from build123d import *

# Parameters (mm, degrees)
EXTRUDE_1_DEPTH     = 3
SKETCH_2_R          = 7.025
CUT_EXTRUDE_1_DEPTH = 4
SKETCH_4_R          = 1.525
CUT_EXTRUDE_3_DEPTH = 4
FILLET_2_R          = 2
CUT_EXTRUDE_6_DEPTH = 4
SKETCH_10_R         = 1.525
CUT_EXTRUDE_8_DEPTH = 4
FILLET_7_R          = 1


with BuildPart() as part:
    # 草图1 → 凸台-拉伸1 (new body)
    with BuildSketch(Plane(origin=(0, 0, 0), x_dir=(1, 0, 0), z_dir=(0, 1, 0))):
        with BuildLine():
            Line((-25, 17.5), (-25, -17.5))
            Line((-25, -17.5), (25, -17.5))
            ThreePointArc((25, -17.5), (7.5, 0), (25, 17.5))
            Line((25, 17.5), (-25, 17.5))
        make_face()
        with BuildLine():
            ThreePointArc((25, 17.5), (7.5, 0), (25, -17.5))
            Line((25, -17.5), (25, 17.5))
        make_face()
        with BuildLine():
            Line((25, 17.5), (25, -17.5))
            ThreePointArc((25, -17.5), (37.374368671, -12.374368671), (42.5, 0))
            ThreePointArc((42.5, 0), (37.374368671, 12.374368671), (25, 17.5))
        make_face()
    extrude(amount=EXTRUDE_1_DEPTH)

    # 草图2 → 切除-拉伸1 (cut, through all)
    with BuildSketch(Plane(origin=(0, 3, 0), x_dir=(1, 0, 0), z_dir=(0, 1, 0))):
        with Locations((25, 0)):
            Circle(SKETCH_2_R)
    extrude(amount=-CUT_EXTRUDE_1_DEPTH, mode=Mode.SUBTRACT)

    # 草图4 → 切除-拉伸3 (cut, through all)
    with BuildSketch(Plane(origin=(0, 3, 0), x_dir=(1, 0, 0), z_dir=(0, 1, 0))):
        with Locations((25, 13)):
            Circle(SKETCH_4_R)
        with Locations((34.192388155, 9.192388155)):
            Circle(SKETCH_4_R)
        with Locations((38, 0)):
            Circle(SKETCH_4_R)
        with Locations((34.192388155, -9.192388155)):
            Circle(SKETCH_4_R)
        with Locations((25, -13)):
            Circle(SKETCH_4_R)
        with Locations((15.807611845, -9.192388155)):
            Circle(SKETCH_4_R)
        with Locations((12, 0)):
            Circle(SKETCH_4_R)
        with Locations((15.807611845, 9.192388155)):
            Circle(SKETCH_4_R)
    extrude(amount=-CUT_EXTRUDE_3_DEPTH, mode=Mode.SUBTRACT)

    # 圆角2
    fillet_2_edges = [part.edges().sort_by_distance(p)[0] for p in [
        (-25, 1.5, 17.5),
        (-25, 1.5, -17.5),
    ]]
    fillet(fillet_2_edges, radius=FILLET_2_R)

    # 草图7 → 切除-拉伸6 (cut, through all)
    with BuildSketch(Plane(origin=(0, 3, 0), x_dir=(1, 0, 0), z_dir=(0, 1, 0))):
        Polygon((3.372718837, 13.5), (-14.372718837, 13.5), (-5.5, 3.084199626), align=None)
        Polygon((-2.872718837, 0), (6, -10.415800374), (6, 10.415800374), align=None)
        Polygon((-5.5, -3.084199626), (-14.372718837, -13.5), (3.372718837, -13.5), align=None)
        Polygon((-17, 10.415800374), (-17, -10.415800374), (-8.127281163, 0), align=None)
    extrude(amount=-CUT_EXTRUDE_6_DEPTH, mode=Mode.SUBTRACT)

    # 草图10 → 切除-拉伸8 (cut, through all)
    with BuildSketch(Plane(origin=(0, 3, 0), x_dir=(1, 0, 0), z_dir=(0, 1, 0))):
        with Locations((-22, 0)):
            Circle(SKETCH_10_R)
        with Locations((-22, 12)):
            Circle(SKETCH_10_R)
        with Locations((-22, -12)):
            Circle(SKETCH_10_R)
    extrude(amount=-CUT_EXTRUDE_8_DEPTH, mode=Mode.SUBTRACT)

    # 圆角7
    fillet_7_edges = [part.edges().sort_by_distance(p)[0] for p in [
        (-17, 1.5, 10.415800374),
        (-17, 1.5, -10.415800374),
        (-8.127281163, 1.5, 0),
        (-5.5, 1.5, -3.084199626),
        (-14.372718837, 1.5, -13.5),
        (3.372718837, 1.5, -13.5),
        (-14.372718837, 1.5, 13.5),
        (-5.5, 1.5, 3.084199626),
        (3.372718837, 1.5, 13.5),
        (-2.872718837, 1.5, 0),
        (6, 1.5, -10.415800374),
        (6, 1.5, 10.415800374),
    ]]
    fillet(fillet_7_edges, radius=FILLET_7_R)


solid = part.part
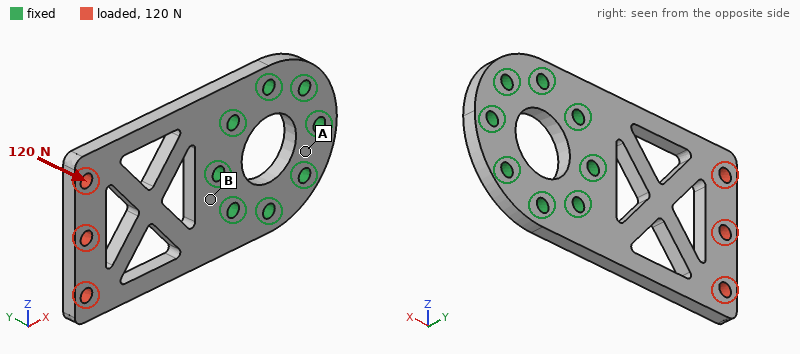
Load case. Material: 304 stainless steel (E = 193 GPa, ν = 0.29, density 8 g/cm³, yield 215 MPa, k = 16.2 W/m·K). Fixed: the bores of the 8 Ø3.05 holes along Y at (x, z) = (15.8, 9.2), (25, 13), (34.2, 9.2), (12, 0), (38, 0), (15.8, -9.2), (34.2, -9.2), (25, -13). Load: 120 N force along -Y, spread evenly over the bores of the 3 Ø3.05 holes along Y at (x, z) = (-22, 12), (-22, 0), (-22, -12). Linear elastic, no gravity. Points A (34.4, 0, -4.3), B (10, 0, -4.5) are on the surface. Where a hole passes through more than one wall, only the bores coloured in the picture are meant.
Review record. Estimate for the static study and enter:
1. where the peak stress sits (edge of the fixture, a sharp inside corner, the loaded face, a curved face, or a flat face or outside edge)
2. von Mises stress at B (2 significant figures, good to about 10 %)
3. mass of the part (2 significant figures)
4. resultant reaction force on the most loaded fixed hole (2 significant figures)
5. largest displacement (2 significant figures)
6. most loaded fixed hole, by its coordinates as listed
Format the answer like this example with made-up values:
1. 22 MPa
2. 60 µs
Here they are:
1. a curved face
2. 59 MPa
3. 39 g
4. 150 N
5. 0.27 mm
6. (12, 0)
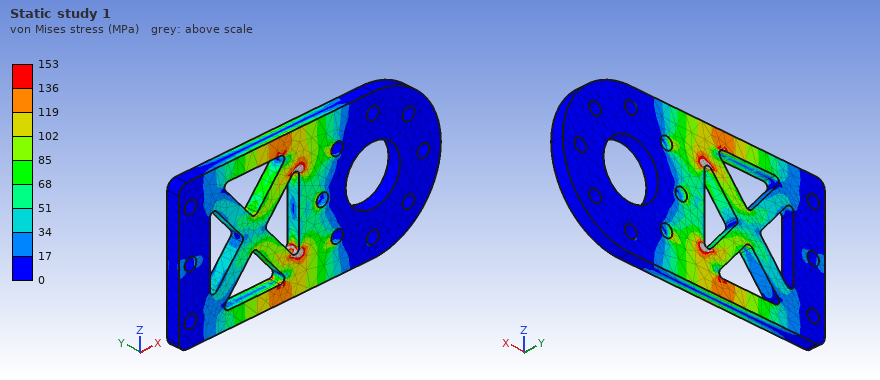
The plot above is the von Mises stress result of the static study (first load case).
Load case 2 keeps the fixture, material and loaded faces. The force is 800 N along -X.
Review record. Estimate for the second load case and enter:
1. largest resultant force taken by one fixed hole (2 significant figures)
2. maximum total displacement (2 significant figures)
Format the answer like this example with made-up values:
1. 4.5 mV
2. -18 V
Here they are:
1. 280 N
2. 9.6 µm
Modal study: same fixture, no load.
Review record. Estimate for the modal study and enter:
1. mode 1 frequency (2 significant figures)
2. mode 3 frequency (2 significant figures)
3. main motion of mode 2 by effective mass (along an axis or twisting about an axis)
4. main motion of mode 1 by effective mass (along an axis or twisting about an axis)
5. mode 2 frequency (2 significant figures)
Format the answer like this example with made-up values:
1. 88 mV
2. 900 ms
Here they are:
1. 1300 Hz
2. 7900 Hz
3. twisting about X
4. along Y
5. 3200 Hz
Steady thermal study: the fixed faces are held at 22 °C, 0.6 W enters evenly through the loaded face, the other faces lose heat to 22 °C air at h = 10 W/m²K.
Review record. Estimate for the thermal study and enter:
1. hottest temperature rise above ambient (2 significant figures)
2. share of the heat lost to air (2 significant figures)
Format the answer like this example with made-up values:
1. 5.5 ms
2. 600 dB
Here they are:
1. 20 K
2. 43 %
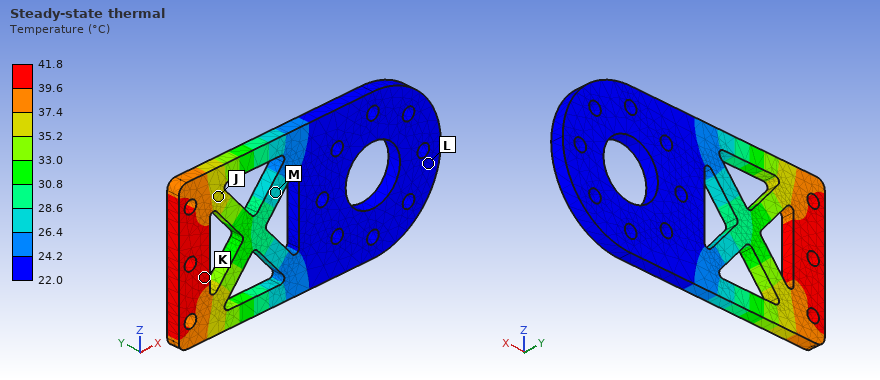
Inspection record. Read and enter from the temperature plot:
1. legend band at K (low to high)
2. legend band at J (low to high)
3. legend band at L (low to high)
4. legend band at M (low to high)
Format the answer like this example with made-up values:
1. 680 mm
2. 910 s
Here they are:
1. 39.6 to 41.8 °C
2. 35.2 to 37.4 °C
3. 22.0 to 24.2 °C
4. 26.4 to 28.6 °C
